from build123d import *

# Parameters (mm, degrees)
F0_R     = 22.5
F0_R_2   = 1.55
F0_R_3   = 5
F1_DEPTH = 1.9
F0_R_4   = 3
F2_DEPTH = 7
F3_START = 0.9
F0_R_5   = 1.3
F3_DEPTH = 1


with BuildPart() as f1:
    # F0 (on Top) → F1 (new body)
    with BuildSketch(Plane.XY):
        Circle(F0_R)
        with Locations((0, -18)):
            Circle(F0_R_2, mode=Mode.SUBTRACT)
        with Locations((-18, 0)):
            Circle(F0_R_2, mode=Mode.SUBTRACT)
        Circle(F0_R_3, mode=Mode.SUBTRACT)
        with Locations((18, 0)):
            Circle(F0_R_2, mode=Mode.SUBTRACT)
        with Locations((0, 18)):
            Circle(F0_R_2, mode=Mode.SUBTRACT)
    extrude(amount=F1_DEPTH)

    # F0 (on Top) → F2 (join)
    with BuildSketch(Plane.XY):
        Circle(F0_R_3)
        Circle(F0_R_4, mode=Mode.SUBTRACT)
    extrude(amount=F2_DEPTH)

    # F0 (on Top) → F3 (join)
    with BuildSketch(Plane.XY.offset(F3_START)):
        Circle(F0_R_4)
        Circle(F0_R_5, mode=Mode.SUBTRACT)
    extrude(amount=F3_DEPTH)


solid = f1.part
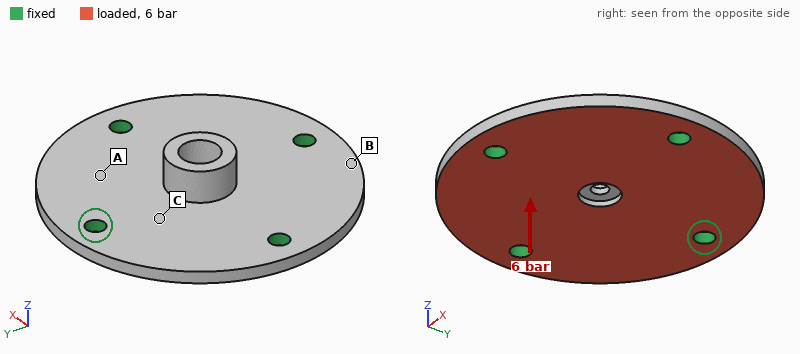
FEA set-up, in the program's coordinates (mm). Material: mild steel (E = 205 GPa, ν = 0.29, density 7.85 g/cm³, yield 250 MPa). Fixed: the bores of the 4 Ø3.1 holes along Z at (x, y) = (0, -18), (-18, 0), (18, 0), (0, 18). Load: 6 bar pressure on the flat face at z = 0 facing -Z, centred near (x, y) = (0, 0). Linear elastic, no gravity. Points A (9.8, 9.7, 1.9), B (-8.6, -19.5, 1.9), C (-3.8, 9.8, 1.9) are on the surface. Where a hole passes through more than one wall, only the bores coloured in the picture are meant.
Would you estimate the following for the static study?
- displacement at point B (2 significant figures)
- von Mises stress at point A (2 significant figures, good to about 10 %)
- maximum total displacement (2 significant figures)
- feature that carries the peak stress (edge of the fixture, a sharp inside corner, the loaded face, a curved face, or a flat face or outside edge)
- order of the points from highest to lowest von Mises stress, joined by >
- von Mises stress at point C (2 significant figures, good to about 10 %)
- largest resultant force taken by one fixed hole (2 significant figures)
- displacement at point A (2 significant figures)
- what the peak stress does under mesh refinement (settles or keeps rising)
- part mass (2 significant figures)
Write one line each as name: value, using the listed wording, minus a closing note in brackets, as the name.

displacement at point B: 4.7 µm
von Mises stress at point A: 30 MPa
maximum total displacement: 9.3 µm
feature that carries the peak stress: edge of the fixture
order of the points from highest to lowest von Mises stress, joined by >: A > C > B
von Mises stress at point C: 22 MPa
largest resultant force taken by one fixed hole: 230 N
displacement at point A: 6.4 µm
what the peak stress does under mesh refinement: keeps rising
part mass: 25 g
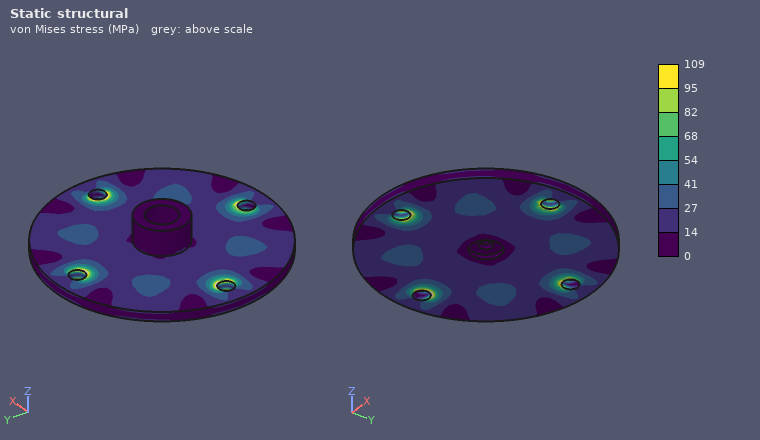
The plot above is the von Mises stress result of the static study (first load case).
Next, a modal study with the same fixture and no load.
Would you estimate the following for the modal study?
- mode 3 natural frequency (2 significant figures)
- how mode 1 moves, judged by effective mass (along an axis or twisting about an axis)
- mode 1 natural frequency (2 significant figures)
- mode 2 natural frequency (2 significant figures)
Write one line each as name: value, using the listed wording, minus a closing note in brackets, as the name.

mode 3 natural frequency: 13 kHz
how mode 1 moves, judged by effective mass: along Z
mode 1 natural frequency: 11 kHz
mode 2 natural frequency: 12 kHz
